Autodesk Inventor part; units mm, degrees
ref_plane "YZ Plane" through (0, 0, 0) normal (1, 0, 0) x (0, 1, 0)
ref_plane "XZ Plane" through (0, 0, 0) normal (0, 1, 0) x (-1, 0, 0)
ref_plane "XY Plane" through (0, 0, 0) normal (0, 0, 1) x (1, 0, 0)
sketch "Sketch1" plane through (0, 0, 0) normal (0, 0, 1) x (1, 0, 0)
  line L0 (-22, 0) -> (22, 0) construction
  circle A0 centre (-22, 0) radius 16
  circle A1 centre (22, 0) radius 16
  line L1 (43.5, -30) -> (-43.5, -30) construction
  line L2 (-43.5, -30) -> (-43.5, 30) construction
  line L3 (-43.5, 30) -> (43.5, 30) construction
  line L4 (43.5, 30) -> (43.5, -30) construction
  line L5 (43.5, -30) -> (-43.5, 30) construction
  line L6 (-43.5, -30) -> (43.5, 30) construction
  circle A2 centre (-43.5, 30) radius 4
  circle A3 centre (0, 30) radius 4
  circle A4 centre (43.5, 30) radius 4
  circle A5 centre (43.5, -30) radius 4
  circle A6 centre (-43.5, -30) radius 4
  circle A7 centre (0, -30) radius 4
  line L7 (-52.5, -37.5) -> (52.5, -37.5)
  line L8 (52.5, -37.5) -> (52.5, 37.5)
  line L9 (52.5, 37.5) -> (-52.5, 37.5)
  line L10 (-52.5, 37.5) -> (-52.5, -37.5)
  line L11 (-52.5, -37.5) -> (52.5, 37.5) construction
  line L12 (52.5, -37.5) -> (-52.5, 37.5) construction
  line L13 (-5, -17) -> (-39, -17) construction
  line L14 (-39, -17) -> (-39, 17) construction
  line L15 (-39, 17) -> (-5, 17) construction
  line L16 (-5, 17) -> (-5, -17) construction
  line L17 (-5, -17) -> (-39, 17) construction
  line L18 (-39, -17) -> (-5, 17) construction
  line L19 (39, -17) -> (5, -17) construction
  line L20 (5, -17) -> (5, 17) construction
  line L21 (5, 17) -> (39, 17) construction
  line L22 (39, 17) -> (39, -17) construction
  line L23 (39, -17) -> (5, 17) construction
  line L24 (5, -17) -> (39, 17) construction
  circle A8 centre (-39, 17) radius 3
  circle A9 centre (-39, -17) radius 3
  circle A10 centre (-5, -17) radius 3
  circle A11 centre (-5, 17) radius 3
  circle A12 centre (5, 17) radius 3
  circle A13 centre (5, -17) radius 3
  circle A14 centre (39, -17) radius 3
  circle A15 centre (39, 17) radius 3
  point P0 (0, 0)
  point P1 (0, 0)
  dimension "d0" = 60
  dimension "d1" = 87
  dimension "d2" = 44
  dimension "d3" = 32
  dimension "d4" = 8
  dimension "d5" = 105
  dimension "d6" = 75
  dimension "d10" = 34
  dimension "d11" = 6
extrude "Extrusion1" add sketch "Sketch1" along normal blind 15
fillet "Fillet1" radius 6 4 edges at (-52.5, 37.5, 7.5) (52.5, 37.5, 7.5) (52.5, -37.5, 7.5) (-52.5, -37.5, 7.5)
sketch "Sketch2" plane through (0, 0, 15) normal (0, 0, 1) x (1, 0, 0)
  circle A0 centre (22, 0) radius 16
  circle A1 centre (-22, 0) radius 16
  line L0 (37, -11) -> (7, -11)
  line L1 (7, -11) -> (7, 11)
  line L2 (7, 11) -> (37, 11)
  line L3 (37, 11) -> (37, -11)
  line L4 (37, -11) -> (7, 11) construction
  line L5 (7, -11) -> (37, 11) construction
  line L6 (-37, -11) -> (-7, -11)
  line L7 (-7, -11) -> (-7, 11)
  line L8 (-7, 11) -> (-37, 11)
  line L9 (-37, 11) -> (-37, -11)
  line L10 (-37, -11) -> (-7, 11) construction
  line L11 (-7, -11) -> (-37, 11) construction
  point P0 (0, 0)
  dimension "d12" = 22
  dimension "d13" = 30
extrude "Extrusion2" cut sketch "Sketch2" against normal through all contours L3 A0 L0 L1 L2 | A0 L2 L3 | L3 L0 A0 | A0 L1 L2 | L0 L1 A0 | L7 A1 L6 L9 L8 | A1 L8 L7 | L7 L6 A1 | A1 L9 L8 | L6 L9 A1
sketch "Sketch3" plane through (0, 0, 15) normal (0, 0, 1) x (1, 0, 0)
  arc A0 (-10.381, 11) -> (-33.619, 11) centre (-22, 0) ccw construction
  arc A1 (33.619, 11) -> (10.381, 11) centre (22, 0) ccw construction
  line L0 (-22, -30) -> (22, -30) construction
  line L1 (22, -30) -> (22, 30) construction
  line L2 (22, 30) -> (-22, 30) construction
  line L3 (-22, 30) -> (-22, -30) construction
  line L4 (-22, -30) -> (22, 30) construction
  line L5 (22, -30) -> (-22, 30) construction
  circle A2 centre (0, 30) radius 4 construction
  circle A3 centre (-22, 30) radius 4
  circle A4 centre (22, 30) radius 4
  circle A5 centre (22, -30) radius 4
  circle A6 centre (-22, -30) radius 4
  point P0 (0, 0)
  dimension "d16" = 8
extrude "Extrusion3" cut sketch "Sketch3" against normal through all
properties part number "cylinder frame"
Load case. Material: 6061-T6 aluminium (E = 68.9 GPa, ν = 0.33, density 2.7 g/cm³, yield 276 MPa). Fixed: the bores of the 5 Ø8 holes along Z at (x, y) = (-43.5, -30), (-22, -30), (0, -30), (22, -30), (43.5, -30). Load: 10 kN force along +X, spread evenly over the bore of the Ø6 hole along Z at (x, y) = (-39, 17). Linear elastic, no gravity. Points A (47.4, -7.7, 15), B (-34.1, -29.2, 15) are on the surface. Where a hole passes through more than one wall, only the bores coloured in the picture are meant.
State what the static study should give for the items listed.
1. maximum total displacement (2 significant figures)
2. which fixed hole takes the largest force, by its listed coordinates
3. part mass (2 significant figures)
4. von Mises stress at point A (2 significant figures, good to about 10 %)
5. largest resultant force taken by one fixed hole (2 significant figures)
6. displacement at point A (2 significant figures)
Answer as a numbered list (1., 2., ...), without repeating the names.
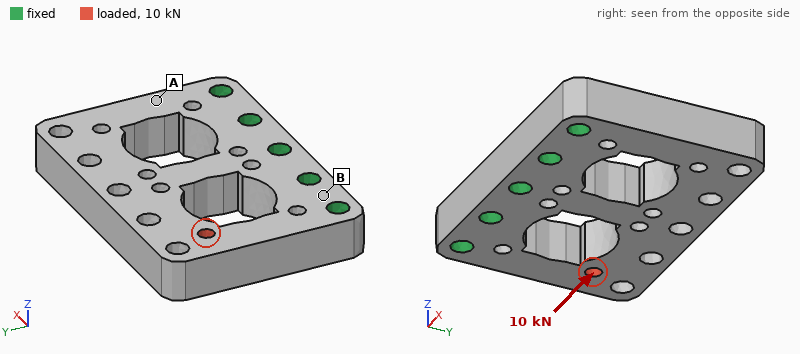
1. 97 µm
2. (-43.5, -30)
3. 220 g
4. 33 MPa
5. 5.5 kN
6. 21 µm
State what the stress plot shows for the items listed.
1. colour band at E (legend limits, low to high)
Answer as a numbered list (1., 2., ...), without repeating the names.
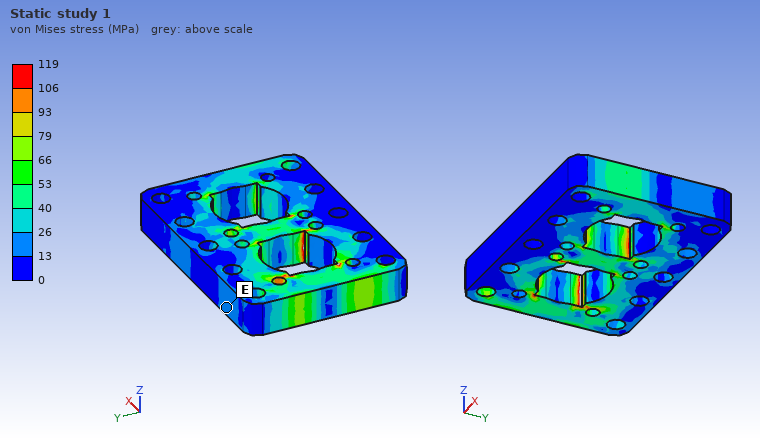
1. 13 to 26 MPa
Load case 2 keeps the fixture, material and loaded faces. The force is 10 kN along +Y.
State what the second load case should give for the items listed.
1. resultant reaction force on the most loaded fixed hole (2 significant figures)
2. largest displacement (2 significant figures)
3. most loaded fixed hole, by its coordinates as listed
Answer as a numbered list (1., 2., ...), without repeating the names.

1. 8.2 kN
2. 34 µm
3. (-43.5, -30)
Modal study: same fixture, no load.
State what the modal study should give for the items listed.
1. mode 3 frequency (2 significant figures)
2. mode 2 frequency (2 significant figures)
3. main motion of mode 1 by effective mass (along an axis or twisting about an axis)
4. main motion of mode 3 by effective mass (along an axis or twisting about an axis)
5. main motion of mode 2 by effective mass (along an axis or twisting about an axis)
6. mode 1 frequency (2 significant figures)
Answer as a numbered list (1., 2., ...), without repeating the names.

1. 5300 Hz
2. 3700 Hz
3. along Z
4. along X
5. twisting about Y
6. 2100 Hz
